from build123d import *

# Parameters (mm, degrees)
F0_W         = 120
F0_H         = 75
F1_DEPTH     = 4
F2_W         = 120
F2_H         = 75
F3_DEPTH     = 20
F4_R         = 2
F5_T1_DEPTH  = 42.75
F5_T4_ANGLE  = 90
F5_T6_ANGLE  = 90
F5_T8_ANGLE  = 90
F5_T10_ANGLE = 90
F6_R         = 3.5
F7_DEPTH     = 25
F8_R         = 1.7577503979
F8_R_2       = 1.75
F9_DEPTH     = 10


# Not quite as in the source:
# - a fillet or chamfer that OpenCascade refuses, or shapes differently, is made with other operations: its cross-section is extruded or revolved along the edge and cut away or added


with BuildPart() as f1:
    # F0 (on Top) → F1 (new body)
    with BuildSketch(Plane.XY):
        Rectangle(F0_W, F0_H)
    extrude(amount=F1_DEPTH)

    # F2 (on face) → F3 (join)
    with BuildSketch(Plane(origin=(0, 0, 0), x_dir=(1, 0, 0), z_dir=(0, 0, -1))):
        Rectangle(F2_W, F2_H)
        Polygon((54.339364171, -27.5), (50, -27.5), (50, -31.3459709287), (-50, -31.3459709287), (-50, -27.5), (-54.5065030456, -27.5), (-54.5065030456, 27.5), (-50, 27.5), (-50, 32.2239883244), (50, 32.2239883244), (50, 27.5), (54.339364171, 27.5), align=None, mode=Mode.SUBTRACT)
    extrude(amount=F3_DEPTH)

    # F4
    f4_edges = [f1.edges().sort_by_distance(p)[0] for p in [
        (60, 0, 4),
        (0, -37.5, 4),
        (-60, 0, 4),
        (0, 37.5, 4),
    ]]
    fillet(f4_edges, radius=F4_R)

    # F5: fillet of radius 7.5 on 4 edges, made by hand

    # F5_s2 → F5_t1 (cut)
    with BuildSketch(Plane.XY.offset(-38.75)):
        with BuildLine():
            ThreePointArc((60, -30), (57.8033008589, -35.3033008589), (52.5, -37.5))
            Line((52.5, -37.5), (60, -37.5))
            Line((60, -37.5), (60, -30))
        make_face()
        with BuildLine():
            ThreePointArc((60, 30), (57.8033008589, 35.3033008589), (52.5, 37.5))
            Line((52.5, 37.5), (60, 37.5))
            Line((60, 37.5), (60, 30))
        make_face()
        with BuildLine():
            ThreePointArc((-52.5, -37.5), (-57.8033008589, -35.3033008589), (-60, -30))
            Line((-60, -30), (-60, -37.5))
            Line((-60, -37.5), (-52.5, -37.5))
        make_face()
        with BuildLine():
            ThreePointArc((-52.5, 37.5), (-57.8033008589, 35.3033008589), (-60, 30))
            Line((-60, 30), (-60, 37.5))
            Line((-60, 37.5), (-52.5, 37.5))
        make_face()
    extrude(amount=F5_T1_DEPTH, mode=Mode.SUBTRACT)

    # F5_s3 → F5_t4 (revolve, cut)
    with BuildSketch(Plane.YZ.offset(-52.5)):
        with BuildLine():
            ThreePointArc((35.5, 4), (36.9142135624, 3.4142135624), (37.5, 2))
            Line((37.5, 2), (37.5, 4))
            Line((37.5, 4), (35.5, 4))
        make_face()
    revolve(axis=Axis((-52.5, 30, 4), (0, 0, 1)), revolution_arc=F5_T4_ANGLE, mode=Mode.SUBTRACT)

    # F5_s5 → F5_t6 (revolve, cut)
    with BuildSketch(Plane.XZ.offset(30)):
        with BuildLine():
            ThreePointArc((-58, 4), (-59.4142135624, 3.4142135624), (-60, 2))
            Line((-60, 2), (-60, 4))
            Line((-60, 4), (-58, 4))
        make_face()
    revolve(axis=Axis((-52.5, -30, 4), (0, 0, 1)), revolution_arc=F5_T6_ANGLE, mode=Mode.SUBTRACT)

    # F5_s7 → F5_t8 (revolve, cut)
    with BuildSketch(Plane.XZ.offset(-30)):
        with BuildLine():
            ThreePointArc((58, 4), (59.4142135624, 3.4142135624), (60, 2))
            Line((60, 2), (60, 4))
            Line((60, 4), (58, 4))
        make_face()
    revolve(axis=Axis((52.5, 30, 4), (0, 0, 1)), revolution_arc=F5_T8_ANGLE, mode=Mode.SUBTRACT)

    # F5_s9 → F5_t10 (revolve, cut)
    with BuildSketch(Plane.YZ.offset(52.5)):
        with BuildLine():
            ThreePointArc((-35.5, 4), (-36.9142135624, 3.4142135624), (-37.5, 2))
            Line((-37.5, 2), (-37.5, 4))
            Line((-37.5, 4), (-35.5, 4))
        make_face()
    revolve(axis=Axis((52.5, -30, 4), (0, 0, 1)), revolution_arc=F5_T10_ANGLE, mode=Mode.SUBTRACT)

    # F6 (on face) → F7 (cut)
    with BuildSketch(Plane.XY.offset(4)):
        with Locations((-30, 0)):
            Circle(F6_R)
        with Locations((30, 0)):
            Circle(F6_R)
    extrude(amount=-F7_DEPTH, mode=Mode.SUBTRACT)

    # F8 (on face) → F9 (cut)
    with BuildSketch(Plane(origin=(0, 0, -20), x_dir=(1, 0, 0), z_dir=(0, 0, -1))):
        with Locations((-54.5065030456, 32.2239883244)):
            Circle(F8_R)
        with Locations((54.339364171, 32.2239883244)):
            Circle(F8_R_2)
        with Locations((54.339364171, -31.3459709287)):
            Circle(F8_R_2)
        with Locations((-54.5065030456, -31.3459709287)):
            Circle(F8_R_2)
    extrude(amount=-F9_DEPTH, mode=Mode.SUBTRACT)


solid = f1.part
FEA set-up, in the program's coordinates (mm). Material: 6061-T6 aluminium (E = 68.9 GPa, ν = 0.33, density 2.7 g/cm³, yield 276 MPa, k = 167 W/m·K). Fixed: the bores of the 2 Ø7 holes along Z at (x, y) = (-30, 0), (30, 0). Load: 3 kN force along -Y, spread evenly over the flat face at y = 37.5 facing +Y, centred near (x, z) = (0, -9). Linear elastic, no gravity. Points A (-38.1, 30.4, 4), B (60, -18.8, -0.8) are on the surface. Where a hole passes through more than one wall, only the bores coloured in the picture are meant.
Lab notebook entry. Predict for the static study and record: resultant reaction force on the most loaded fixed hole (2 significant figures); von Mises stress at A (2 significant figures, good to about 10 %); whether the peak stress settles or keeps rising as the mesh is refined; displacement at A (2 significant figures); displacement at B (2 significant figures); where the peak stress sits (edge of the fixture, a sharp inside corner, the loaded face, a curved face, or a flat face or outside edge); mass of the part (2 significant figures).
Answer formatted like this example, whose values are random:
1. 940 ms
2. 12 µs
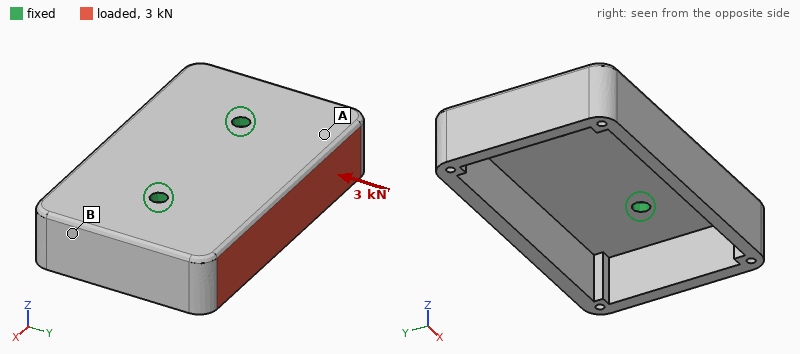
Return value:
1. 1.5 kN
2. 31 MPa
3. keeps rising
4. 0.19 mm
5. 0.11 mm
6. edge of the fixture
7. 210 g
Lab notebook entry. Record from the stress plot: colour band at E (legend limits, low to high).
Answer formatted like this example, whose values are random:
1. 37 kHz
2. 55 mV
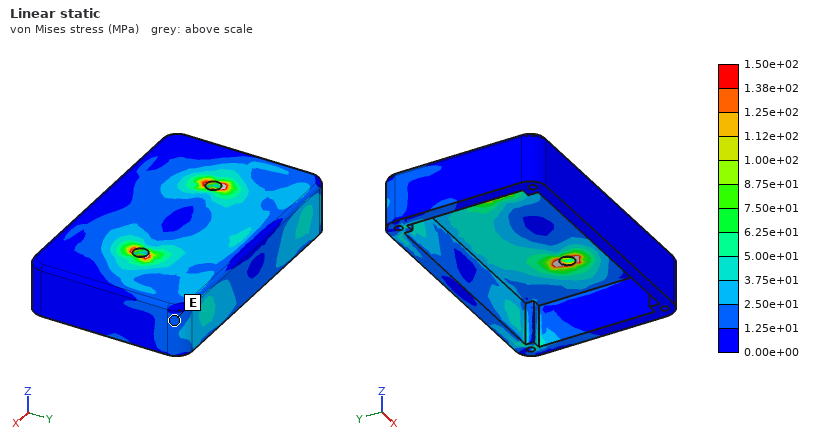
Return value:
1. 1.25e+01 to 2.50e+01 MPa
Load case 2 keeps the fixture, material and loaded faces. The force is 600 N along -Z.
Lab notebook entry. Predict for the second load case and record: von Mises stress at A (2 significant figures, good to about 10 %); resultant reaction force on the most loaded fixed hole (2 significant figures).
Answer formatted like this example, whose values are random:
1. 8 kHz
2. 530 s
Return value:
1. 15 MPa
2. 310 N
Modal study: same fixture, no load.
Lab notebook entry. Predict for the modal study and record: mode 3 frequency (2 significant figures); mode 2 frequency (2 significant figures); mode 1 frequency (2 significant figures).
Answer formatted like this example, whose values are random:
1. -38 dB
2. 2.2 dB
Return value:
1. 1800 Hz
2. 1600 Hz
3. 970 Hz
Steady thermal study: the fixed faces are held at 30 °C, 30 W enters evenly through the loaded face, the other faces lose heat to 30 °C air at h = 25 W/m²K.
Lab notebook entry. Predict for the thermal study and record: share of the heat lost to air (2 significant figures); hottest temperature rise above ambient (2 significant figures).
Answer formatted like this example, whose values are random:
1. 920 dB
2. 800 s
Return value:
1. 17 %
2. 16 K
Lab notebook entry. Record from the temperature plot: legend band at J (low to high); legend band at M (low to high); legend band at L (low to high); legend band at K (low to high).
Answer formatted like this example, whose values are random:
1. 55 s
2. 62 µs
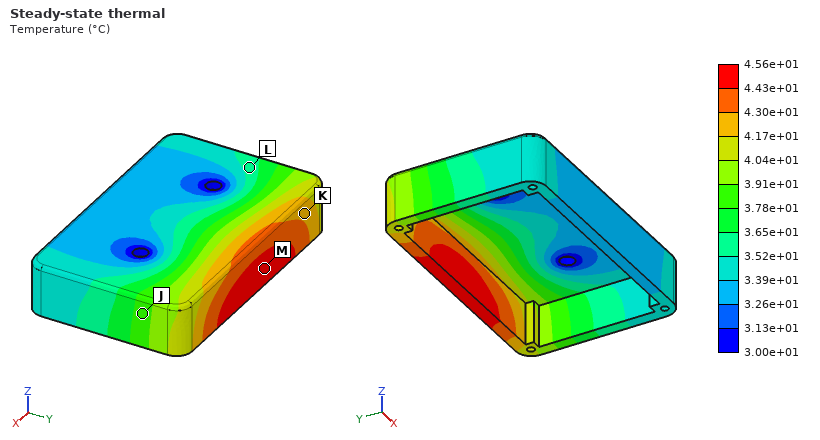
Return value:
1. 3.78e+01 to 3.91e+01 °C
2. 4.43e+01 to 4.56e+01 °C
3. 3.52e+01 to 3.65e+01 °C
4. 4.17e+01 to 4.30e+01 °C
